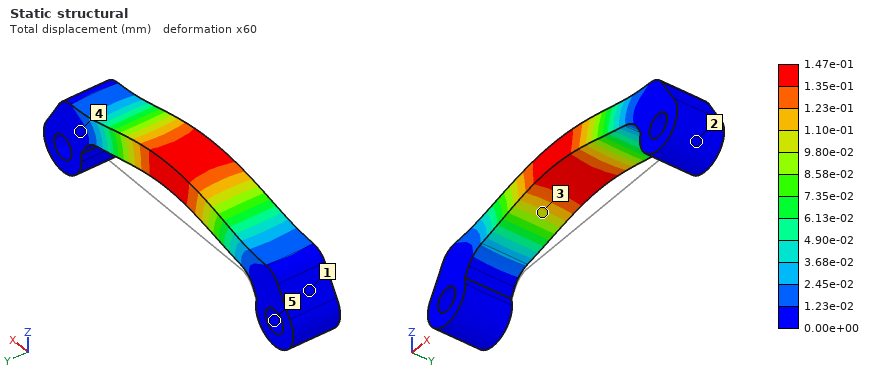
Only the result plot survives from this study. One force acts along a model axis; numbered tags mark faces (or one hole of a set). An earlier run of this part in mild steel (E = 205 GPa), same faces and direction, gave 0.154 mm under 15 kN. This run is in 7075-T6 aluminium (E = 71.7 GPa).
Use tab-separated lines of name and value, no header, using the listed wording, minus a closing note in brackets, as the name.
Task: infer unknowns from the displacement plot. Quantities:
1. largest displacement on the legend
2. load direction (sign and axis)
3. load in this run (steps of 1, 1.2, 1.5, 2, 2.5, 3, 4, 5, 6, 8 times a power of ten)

largest displacement on the legend	1.47e-01 mm
load direction	+Z
load in this run	5 kN
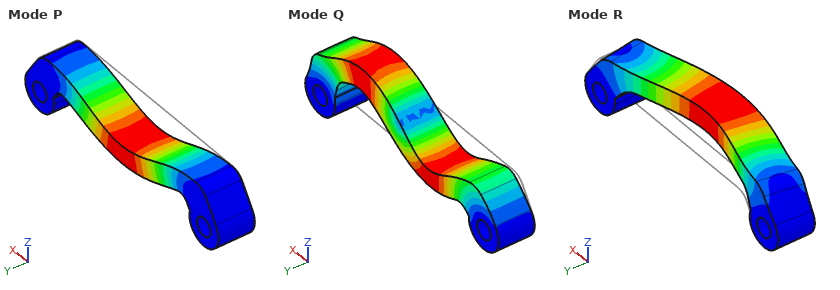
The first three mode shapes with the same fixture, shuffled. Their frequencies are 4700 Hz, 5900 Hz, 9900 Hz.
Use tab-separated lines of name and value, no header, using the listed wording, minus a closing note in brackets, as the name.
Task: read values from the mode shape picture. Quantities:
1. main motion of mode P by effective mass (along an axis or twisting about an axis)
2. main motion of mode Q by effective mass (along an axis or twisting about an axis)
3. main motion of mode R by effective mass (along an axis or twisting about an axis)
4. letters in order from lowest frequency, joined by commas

main motion of mode P by effective mass	along Z
main motion of mode Q by effective mass	along X
main motion of mode R by effective mass	along Y
letters in order from lowest frequency, joined by commas	P, R, Q
